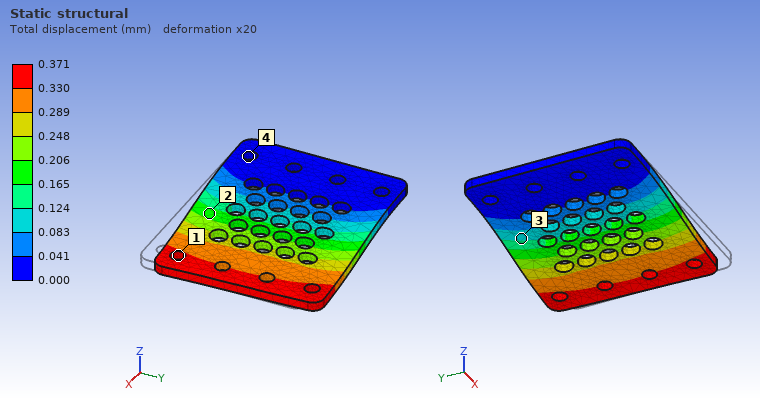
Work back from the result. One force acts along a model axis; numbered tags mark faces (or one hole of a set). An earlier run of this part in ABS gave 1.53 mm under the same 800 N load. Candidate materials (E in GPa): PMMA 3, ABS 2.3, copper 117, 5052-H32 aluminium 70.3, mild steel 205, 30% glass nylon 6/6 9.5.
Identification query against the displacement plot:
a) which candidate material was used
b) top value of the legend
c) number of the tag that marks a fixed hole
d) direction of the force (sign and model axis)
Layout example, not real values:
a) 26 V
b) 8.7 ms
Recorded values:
a) 30% glass nylon 6/6
b) 0.371 mm
c) 4
d) +Y
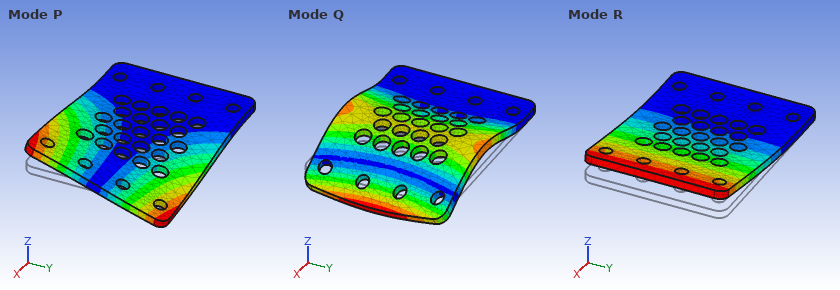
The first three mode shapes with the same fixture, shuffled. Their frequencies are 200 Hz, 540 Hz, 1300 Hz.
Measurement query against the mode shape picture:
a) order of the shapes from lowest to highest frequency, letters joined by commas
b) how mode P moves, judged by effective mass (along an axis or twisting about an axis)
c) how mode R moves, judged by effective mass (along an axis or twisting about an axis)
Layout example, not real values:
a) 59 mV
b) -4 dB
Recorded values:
a) R, P, Q
b) twisting about X
c) along Z
